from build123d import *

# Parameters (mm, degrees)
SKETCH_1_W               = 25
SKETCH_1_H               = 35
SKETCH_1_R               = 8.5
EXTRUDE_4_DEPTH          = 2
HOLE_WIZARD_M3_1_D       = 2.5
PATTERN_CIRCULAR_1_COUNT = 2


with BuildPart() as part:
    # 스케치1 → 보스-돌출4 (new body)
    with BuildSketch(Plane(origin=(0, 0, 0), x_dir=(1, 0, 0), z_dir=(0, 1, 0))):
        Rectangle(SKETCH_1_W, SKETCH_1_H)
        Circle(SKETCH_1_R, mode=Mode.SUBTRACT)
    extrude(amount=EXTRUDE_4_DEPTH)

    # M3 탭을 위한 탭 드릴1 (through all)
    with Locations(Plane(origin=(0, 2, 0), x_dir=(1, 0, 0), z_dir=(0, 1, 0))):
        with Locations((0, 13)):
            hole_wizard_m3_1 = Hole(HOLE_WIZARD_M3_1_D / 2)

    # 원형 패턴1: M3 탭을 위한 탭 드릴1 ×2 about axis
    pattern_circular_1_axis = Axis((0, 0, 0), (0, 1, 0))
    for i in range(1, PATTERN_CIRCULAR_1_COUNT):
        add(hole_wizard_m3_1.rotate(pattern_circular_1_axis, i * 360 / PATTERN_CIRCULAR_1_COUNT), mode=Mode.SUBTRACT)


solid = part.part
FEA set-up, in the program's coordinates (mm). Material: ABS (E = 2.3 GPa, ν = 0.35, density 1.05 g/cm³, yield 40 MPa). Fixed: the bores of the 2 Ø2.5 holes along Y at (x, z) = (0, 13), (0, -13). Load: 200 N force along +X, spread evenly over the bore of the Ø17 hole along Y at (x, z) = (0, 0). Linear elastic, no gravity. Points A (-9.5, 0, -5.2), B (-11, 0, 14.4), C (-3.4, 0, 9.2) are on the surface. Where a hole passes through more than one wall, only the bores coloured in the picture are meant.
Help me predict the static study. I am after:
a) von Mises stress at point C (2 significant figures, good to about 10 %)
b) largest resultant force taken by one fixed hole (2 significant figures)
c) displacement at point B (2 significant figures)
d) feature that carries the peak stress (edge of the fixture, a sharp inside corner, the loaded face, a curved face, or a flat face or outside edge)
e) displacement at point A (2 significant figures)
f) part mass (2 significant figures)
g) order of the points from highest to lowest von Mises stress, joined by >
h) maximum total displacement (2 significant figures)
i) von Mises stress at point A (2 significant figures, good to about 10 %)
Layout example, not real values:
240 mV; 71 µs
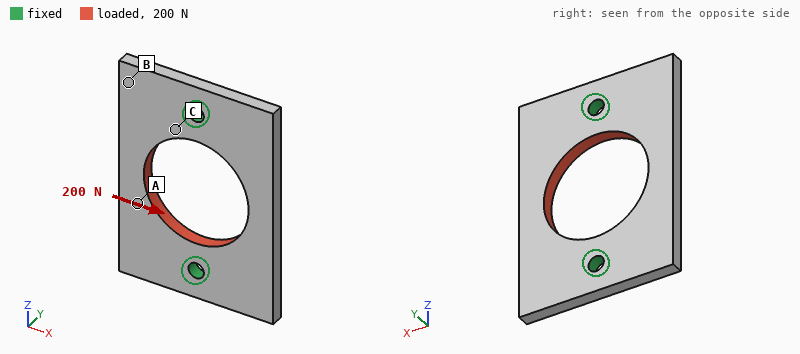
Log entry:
6.0 MPa; 100 N; 14 µm; edge of the fixture; 37 µm; 1.3 g; C > A > B; 55 µm; 4.2 MPa
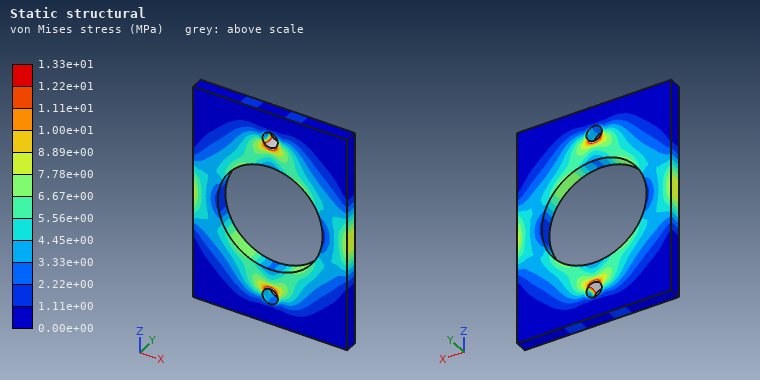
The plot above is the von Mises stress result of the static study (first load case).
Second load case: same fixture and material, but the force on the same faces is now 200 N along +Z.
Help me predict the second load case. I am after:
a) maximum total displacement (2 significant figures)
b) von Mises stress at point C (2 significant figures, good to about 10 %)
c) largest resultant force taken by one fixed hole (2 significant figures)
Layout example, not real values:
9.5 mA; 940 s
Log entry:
48 µm; 5.3 MPa; 100 N
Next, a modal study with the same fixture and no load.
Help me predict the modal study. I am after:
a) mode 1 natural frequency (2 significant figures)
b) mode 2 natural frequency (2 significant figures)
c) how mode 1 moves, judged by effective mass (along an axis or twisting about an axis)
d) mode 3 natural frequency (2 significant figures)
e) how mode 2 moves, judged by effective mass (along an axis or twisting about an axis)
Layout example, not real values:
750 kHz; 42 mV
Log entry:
2200 Hz; 2300 Hz; twisting about Z; 3500 Hz; along Y
